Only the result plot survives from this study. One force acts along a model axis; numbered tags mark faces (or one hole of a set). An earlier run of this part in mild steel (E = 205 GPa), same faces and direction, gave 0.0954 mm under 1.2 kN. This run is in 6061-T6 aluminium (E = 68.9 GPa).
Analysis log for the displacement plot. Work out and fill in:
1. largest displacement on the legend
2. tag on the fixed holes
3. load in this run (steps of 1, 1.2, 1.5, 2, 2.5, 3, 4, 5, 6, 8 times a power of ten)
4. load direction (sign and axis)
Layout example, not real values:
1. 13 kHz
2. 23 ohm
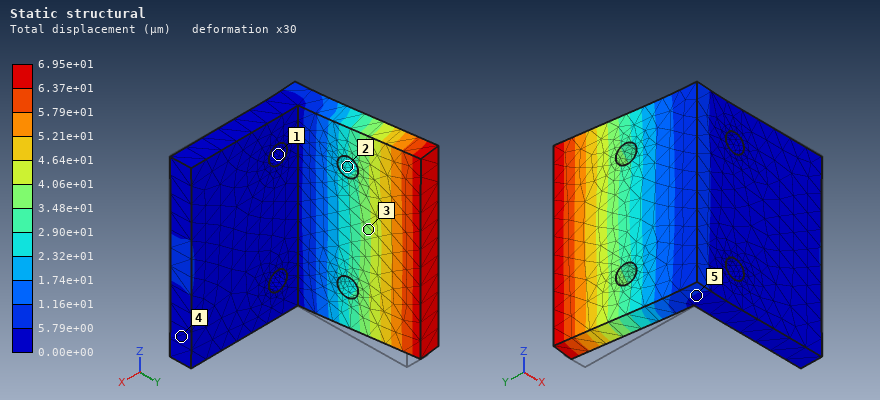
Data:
1. 6.95e+01 µm
2. 1
3. 300 N
4. -X
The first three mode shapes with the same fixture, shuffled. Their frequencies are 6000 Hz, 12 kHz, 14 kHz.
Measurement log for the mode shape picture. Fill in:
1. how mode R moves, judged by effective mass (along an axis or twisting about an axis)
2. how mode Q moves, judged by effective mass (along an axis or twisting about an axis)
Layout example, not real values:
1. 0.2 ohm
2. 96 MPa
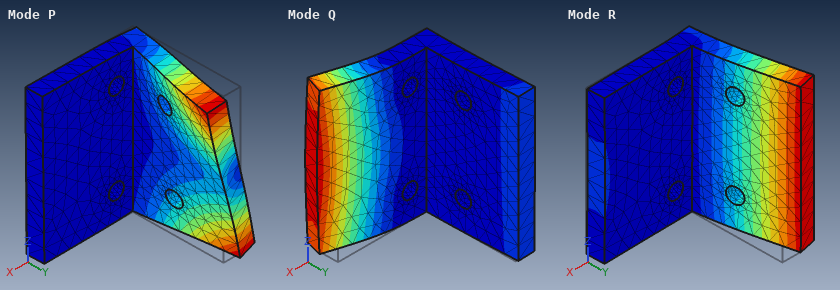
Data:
1. along X
2. along Y
